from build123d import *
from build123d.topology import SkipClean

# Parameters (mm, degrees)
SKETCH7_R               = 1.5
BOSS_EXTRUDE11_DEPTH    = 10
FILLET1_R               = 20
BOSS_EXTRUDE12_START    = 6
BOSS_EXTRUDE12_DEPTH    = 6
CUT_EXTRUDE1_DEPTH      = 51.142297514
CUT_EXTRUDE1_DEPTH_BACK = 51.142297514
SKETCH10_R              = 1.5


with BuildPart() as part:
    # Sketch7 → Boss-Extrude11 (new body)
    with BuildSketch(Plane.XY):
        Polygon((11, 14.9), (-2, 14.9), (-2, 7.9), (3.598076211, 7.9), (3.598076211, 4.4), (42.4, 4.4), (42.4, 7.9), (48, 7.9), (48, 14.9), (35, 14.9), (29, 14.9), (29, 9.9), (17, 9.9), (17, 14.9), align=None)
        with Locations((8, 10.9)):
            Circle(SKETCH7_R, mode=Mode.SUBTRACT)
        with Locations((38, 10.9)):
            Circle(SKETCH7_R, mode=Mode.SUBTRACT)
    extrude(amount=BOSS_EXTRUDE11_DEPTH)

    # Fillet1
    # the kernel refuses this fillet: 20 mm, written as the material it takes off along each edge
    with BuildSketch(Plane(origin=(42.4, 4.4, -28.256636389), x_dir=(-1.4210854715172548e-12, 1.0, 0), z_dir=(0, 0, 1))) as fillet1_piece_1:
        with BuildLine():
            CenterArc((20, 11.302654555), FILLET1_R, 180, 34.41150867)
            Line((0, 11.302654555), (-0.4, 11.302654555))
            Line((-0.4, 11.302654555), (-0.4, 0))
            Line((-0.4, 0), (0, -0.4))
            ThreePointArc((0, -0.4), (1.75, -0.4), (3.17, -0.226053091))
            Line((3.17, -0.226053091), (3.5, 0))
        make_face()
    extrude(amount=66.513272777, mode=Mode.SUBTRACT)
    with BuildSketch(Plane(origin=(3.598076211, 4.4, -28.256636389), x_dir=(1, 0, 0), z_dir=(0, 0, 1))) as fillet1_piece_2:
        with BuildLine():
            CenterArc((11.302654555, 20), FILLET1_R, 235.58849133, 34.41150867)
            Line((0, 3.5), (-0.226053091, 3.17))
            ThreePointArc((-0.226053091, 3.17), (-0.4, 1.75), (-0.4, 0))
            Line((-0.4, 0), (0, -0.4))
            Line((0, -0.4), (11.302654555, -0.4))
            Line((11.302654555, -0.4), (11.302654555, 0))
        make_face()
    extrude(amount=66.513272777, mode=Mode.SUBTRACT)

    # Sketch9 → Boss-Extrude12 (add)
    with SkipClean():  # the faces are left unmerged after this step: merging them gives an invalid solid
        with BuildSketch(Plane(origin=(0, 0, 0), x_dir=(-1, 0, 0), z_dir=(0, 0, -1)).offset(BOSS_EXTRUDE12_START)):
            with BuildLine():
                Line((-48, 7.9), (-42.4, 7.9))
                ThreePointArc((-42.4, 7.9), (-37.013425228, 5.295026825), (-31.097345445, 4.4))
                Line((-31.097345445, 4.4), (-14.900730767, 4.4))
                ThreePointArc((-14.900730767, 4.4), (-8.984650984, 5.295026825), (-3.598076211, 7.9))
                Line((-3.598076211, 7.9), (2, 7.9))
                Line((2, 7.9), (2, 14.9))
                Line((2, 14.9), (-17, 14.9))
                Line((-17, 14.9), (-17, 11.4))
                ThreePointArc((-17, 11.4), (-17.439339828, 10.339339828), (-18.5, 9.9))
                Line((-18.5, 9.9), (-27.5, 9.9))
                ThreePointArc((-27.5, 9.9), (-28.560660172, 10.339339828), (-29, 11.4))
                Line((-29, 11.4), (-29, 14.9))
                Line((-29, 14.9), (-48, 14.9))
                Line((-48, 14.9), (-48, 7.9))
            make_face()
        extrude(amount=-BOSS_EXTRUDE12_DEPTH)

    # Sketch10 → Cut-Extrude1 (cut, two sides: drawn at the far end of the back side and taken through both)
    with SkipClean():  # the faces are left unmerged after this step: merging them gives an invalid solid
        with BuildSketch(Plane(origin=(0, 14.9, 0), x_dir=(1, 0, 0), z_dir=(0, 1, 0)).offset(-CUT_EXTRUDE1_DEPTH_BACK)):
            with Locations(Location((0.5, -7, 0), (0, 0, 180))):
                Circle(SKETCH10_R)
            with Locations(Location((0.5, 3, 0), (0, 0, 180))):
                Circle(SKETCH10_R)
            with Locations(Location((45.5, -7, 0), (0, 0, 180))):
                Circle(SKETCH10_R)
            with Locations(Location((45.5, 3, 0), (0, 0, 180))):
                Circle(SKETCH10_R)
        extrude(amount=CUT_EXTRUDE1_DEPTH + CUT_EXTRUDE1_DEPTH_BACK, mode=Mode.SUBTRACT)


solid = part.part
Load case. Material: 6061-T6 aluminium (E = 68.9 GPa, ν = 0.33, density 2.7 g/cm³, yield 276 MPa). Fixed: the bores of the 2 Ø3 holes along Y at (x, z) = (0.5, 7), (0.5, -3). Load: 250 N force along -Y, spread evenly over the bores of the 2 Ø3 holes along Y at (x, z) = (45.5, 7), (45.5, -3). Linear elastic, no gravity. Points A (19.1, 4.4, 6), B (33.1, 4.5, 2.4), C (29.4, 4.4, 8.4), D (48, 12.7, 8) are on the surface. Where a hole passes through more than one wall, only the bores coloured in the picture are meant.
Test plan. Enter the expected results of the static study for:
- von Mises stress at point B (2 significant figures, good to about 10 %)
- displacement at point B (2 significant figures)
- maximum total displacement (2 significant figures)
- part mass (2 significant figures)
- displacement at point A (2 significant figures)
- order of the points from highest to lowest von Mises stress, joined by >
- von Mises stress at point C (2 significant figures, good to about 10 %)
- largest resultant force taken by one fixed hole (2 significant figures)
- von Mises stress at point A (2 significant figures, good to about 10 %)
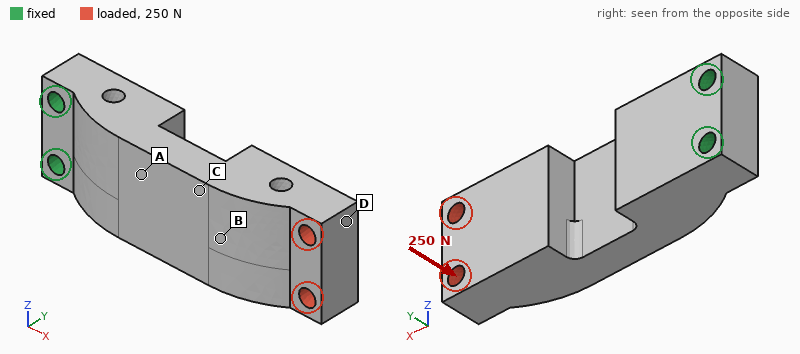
20 MPa
0.15 mm
0.28 mm
16 g
0.050 mm
A > C > B > D
40 MPa
130 N
72 MPa
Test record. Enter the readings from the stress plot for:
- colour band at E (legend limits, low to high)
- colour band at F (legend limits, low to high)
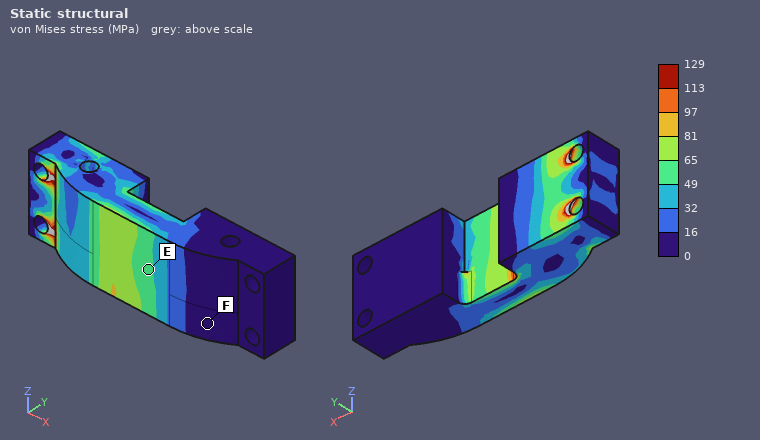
49 to 65 MPa
0 to 16 MPa
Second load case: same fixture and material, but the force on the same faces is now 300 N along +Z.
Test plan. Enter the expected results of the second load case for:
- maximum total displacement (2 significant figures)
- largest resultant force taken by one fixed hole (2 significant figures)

85 µm
1.2 kN
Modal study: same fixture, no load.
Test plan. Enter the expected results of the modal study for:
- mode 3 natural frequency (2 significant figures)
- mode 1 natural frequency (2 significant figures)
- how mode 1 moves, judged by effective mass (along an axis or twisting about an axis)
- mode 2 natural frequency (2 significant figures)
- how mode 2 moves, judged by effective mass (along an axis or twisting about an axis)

11 kHz
2500 Hz
along Y
4900 Hz
along Z
